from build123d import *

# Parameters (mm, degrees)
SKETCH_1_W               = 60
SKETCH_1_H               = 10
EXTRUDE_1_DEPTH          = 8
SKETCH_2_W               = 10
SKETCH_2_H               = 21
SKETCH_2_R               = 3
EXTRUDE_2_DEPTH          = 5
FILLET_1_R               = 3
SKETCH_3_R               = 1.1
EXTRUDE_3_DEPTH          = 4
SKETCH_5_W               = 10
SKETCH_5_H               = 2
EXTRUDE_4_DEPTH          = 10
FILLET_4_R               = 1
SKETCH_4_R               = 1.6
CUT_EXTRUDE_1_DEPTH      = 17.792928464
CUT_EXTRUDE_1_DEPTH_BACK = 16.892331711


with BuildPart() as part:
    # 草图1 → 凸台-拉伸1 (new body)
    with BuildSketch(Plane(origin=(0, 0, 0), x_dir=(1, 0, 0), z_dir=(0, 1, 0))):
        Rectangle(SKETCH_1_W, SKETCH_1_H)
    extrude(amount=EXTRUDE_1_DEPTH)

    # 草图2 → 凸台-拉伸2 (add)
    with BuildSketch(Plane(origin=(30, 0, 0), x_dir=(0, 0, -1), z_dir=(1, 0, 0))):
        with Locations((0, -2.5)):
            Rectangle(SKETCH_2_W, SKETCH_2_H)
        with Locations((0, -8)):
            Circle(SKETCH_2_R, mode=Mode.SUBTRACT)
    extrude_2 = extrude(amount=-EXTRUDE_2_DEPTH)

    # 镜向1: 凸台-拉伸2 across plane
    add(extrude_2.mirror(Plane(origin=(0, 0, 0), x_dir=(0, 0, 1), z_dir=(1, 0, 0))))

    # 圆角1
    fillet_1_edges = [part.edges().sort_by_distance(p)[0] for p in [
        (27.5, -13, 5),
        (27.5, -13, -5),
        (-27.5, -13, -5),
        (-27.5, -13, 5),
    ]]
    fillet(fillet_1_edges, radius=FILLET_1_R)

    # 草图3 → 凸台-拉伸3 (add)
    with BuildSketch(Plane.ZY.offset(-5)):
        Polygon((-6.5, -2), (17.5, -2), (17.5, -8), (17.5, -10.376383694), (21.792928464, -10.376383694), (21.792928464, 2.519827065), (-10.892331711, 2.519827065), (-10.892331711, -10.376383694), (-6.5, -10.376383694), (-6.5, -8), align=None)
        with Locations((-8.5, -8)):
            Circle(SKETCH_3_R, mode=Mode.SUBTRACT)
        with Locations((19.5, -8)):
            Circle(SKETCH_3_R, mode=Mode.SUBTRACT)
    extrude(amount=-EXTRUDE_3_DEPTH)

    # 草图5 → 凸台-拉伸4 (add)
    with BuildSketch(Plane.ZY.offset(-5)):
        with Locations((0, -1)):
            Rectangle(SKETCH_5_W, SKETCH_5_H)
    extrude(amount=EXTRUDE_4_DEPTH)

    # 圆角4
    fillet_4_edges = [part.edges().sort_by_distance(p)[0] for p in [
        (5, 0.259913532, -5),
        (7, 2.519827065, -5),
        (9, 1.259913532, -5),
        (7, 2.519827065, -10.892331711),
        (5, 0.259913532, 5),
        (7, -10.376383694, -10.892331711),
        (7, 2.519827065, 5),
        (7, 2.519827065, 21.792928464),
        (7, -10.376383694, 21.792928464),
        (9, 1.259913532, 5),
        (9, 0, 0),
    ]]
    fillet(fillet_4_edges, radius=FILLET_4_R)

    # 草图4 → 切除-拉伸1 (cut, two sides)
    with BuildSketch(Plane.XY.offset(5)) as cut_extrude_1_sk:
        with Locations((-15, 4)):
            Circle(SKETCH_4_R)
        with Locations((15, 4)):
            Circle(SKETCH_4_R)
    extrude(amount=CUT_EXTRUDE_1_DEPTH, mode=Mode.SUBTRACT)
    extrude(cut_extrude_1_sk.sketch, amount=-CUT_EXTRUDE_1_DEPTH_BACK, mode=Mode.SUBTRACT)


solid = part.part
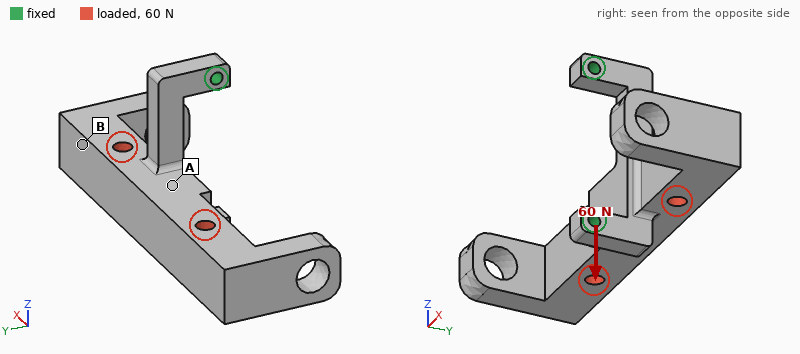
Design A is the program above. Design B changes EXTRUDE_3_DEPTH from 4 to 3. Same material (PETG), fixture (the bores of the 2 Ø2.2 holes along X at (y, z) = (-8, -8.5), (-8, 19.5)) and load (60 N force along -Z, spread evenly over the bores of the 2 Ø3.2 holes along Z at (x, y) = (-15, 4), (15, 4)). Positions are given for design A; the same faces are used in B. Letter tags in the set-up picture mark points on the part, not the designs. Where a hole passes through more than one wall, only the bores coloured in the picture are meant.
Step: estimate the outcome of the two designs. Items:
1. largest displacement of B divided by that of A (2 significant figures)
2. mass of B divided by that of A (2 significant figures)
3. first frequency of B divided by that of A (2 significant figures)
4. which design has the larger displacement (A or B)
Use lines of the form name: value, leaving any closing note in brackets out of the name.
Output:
largest displacement of B divided by that of A: 1.7
mass of B divided by that of A: 0.97
first frequency of B divided by that of A: 0.70
which design has the larger displacement: B
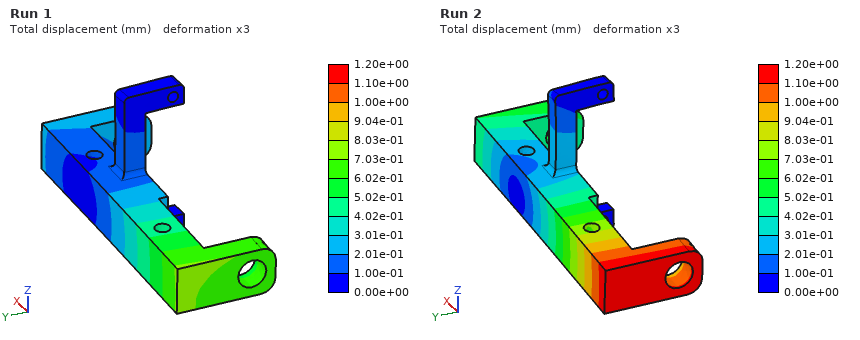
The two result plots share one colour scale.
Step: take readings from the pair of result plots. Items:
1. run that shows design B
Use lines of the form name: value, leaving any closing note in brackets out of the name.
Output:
run that shows design B: Run 2
